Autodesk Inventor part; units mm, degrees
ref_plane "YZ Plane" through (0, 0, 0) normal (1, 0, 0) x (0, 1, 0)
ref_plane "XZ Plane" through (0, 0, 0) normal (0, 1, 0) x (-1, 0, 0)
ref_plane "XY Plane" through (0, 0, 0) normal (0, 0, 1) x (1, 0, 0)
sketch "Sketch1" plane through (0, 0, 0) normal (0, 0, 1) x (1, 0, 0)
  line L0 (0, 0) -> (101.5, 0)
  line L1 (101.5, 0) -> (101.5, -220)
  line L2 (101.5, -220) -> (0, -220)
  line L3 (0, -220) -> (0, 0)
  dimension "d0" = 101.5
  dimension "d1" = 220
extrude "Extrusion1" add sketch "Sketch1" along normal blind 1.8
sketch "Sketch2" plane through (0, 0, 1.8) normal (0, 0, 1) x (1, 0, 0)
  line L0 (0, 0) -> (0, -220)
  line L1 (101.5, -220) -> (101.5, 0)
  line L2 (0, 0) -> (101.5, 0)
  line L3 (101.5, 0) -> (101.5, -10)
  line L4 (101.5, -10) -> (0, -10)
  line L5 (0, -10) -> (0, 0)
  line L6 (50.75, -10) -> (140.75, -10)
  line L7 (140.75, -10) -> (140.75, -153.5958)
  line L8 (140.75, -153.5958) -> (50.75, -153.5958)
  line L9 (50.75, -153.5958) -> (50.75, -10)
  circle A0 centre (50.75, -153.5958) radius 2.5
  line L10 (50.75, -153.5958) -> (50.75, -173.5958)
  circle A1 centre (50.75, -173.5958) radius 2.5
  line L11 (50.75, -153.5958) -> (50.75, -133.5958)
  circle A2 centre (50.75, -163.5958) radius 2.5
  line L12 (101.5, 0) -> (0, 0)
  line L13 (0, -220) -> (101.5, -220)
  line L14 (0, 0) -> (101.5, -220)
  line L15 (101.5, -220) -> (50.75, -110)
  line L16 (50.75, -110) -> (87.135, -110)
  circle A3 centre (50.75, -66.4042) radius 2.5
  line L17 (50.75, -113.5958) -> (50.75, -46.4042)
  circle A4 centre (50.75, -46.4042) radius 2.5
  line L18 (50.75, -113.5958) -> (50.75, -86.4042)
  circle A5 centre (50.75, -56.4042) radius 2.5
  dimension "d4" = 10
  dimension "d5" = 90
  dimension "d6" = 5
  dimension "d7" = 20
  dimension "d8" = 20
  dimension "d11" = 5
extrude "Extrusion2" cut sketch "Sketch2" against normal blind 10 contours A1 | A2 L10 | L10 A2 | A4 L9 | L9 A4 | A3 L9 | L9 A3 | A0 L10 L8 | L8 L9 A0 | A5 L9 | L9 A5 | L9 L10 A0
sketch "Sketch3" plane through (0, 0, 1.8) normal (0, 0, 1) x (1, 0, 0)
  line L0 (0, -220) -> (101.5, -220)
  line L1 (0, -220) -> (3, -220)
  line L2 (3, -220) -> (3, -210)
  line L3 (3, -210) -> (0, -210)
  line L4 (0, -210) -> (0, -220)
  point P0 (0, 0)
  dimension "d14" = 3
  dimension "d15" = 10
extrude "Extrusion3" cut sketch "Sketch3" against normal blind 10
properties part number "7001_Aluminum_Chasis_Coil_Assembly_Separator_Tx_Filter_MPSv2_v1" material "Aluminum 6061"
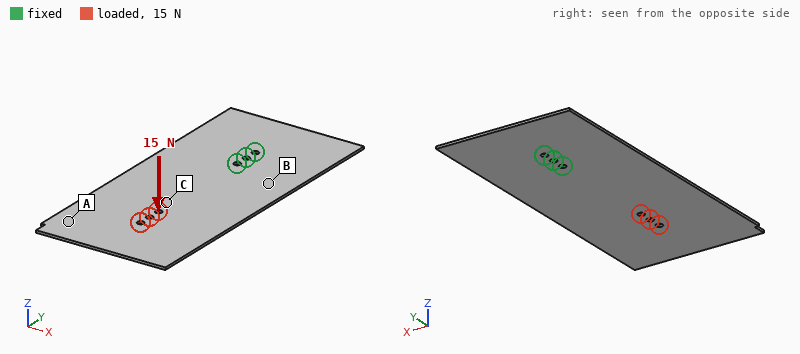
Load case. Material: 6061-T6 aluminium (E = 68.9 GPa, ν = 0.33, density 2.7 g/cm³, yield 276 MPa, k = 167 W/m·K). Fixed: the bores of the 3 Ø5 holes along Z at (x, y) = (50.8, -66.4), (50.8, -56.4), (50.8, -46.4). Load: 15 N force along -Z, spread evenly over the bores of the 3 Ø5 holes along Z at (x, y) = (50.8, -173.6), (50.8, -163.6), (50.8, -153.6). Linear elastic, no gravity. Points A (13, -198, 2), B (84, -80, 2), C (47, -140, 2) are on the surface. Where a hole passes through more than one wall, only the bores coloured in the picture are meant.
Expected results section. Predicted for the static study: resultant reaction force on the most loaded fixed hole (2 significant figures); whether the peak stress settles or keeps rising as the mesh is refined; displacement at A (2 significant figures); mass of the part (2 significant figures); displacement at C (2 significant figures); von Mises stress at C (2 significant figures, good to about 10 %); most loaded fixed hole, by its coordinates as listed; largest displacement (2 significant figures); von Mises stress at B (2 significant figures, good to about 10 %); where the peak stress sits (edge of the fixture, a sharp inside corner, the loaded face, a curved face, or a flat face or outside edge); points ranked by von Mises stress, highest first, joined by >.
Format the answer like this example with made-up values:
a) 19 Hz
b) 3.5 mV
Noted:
a) 64 N
b) keeps rising
c) 2.3 mm
d) 110 g
e) 1.0 mm
f) 6.8 MPa
g) (50.8, -66.4)
h) 2.8 mm
i) 19 MPa
j) edge of the fixture
k) B > C > A
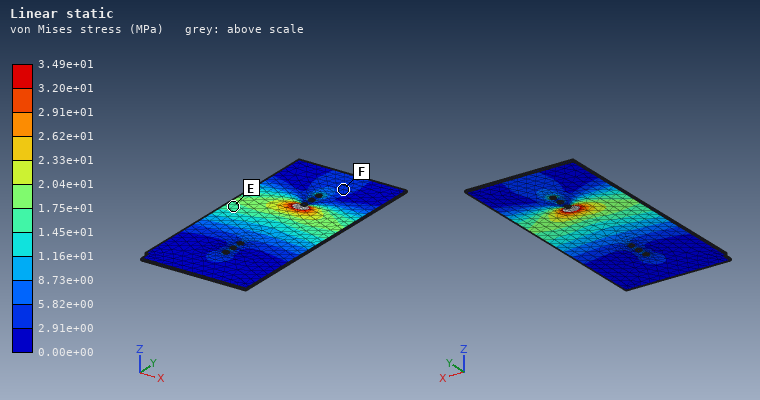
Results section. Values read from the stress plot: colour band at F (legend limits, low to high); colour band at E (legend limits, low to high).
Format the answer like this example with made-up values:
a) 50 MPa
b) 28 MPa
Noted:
a) 2.91e+00 to 5.82e+00 MPa
b) 1.45e+01 to 1.75e+01 MPa
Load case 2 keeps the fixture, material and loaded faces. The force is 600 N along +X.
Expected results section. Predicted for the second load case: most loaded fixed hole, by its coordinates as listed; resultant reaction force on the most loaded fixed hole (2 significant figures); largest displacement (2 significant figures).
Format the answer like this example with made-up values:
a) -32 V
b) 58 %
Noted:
a) (50.8, -66.4)
b) 2.9 kN
c) 0.30 mm
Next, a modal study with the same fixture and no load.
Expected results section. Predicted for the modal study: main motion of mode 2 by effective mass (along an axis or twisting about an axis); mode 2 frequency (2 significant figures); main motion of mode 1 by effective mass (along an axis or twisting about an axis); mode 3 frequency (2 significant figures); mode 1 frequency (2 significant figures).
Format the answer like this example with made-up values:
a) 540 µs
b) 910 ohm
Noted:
a) twisting about Y
b) 170 Hz
c) along Z
d) 350 Hz
e) 60 Hz
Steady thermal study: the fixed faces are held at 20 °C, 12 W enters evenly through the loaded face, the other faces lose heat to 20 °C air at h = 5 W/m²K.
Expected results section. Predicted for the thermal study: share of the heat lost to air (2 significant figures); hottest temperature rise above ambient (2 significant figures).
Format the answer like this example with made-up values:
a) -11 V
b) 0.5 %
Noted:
a) 34 %
b) 41 K
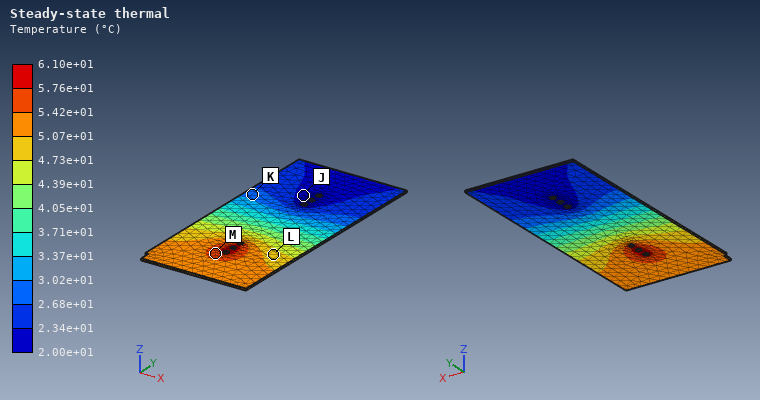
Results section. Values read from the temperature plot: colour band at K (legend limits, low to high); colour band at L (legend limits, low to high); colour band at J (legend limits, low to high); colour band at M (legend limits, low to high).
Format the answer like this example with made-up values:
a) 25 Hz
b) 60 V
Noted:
a) 2.68e+01 to 3.02e+01 °C
b) 4.73e+01 to 5.07e+01 °C
c) 2.00e+01 to 2.34e+01 °C
d) 5.42e+01 to 5.76e+01 °C
